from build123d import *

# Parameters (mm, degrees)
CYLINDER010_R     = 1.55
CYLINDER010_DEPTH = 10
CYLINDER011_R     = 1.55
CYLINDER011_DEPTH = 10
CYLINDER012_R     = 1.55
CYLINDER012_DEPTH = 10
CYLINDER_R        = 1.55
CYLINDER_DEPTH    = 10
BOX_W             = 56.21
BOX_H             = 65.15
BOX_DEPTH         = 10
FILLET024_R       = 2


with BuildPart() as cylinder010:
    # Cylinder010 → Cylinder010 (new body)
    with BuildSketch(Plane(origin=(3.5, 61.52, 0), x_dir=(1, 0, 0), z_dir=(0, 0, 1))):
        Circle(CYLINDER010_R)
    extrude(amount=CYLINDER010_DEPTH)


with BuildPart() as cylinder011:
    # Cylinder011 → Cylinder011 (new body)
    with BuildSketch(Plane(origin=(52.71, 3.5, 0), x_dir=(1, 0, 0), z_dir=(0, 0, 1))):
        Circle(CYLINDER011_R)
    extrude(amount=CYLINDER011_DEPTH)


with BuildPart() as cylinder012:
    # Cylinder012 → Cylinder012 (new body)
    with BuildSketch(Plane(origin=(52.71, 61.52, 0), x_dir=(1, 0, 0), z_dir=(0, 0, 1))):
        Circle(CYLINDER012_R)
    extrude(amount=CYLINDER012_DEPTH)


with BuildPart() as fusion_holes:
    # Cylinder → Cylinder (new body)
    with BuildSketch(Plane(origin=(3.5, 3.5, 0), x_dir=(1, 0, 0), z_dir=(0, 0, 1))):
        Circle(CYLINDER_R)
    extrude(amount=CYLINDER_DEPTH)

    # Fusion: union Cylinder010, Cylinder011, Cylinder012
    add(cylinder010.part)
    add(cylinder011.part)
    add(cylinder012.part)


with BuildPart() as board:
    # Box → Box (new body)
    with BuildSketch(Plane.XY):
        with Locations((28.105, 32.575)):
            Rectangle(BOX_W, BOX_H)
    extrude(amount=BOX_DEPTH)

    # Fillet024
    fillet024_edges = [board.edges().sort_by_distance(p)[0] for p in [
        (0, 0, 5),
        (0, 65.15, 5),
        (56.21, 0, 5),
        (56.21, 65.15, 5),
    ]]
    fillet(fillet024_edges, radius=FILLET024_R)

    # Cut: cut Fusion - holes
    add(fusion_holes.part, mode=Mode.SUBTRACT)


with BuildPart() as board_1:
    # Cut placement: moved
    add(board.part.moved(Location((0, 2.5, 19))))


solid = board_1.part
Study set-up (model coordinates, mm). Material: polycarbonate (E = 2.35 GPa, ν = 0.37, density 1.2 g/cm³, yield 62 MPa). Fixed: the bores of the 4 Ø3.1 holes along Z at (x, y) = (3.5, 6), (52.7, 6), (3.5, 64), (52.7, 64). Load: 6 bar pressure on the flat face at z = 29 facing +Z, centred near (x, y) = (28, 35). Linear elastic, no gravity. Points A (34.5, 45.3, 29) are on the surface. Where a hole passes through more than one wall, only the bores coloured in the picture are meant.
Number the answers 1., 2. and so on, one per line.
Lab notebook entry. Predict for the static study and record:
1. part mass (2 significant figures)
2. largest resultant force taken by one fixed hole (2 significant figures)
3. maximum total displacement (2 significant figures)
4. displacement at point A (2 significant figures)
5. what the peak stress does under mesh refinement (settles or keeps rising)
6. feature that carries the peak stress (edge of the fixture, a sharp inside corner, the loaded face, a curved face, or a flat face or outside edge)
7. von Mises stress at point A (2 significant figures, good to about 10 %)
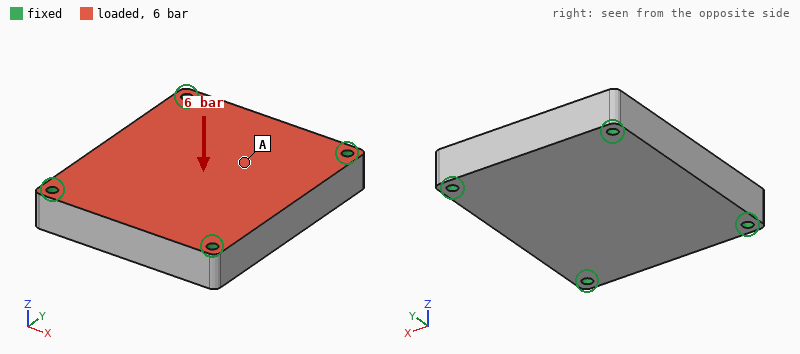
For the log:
1. 44 g
2. 550 N
3. 0.27 mm
4. 0.24 mm
5. keeps rising
6. edge of the fixture
7. 5.3 MPa
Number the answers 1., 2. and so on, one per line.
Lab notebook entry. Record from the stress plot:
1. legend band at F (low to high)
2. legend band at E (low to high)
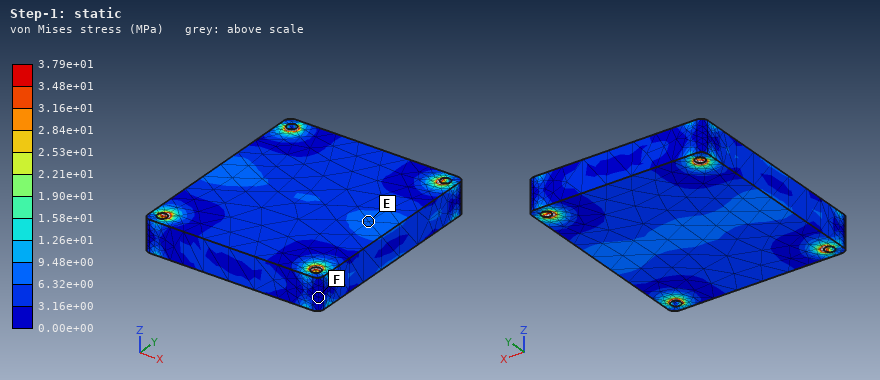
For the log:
1. 0.00e+00 to 3.16e+00 MPa
2. 6.32e+00 to 9.48e+00 MPa
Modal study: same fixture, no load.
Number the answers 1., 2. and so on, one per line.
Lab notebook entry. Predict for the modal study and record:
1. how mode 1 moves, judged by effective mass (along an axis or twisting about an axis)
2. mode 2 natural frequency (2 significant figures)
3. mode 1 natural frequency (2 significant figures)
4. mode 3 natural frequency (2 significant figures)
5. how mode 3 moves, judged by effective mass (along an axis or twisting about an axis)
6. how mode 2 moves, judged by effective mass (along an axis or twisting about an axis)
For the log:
1. along Z
2. 3900 Hz
3. 2500 Hz
4. 4500 Hz
5. twisting about X
6. twisting about Y
